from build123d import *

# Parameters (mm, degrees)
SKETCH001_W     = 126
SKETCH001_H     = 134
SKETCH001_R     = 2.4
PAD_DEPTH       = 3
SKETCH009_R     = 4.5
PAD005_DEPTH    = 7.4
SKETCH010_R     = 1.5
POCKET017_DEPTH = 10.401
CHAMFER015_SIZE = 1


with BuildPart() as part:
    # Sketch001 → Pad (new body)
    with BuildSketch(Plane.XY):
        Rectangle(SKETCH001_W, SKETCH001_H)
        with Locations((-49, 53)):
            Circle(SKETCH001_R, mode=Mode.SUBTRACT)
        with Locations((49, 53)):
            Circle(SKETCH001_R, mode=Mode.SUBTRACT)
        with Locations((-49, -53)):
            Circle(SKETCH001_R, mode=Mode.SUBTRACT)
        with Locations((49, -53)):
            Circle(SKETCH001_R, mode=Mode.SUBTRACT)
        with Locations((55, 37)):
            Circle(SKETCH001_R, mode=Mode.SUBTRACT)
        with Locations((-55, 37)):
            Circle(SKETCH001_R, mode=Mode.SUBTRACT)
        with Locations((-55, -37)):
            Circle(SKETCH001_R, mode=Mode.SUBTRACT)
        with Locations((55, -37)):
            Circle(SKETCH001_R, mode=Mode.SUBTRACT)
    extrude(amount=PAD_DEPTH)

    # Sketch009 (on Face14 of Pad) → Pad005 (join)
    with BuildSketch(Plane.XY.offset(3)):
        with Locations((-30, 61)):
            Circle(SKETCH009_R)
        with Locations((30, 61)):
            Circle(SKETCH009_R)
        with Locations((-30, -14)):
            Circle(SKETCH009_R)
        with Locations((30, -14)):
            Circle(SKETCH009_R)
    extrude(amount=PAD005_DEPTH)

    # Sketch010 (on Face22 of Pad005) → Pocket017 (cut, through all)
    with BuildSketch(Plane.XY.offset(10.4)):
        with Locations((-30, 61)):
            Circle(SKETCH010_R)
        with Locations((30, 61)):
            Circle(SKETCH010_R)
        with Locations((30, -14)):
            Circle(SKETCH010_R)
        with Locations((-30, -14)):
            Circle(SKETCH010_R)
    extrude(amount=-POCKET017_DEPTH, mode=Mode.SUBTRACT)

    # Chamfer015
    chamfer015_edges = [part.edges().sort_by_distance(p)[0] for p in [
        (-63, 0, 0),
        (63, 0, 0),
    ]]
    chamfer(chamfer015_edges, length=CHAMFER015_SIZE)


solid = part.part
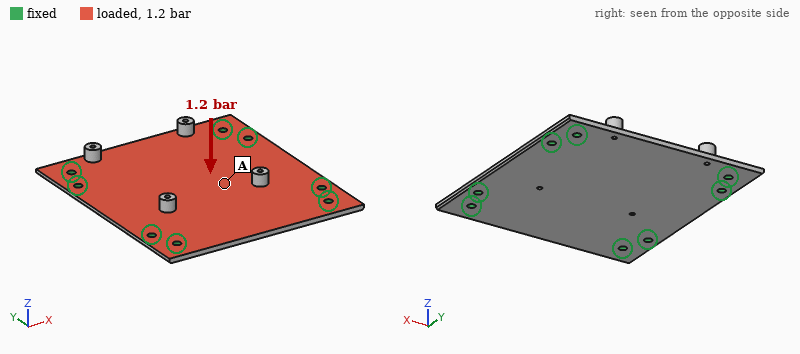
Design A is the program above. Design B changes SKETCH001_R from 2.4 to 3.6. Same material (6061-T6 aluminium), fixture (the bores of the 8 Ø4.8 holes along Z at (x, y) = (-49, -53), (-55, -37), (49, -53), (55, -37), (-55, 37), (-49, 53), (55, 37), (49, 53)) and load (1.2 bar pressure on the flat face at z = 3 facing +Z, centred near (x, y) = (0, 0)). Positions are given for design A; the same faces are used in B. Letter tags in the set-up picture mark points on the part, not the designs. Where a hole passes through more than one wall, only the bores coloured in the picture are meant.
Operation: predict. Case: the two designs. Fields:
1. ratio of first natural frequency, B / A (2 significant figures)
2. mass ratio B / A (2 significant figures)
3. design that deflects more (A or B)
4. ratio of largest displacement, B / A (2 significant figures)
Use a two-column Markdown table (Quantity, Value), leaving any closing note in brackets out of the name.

| Quantity | Value |
|---|---|
| ratio of first natural frequency, B / A | 1.1 |
| mass ratio B / A | 0.99 |
| design that deflects more | A |
| ratio of largest displacement, B / A | 0.89 |
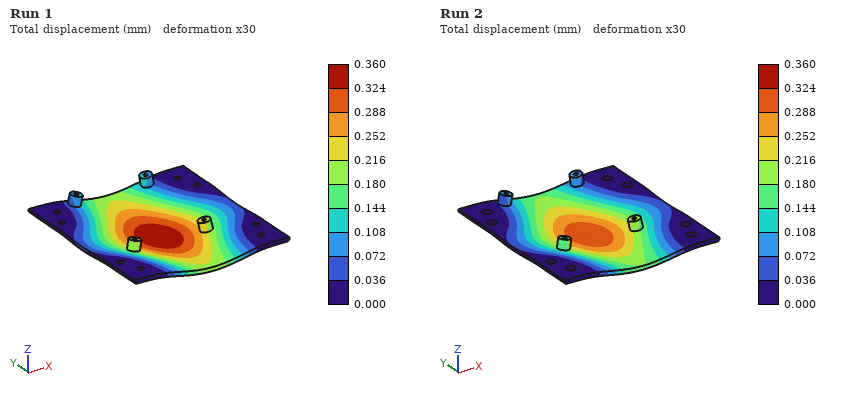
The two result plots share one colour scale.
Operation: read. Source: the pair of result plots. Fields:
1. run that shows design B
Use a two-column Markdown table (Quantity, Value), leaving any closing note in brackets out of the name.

| Quantity | Value |
|---|---|
| run that shows design B | Run 2 |
